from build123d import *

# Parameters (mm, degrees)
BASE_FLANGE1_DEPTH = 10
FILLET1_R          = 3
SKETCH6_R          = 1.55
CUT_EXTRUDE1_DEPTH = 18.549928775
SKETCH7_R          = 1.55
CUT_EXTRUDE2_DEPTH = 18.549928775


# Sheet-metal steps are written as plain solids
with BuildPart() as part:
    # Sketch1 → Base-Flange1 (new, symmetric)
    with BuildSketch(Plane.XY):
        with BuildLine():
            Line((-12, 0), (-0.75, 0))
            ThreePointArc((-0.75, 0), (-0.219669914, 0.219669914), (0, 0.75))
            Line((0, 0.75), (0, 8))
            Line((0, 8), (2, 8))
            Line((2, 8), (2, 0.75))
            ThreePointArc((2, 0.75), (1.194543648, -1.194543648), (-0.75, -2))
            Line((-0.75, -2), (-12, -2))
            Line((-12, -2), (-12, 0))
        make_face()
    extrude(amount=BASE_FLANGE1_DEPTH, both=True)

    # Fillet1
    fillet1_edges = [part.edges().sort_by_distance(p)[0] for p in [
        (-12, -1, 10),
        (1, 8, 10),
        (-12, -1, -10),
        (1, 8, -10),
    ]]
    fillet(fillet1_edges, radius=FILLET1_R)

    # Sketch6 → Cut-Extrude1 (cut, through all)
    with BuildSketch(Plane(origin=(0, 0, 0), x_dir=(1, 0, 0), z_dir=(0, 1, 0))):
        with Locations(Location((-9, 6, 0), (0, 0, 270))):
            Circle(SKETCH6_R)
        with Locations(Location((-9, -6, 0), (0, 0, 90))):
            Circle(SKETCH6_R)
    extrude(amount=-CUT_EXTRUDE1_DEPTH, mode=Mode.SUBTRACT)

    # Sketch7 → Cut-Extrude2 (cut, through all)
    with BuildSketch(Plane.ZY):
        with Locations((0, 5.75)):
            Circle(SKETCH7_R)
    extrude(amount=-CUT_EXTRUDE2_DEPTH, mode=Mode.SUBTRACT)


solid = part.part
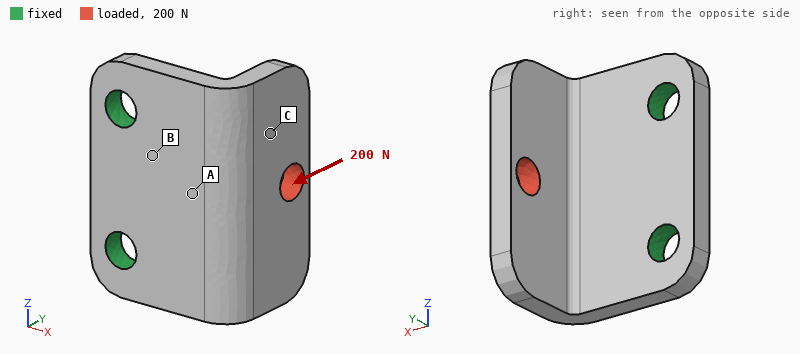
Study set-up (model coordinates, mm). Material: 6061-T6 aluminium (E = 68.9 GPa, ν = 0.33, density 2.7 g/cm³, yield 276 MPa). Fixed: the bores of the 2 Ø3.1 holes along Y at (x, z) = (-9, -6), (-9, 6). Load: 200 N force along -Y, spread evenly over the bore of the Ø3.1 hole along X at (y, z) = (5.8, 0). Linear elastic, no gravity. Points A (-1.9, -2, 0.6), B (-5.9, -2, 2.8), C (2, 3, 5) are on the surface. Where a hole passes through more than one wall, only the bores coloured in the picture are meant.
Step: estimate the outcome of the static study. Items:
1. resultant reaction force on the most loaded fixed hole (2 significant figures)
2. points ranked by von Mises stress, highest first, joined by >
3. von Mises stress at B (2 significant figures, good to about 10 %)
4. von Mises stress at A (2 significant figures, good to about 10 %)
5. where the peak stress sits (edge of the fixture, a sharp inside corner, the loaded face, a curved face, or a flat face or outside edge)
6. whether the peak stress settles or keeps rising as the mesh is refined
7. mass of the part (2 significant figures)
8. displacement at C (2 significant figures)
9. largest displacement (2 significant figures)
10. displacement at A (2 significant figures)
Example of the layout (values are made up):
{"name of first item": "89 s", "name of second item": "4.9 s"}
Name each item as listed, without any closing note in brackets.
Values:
{"resultant reaction force on the most loaded fixed hole": "100 N", "points ranked by von Mises stress, highest first, joined by >": "B > A > C", "von Mises stress at B": "77 MPa", "von Mises stress at A": "41 MPa", "where the peak stress sits": "edge of the fixture", "whether the peak stress settles or keeps rising as the mesh is refined": "keeps rising", "mass of the part": "2.1 g", "displacement at C": "0.077 mm", "largest displacement": "0.11 mm", "displacement at A": "0.035 mm"}
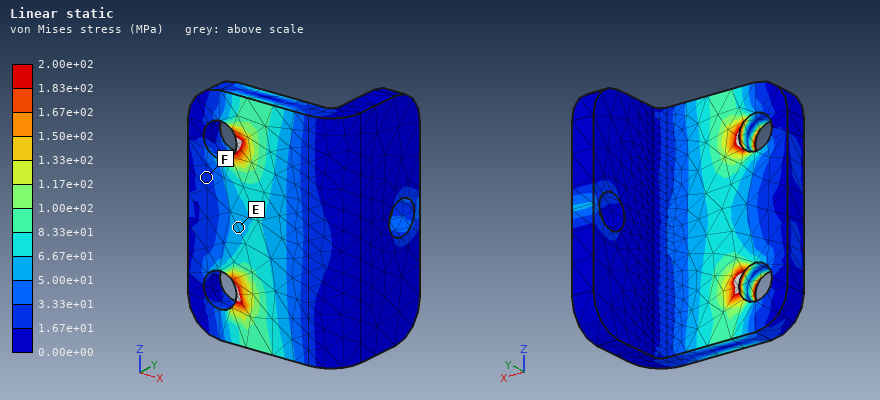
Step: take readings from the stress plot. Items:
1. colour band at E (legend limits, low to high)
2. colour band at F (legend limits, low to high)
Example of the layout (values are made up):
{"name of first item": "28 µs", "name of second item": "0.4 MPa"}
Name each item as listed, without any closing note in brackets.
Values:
{"colour band at E": "5.00e+01 to 6.67e+01 MPa", "colour band at F": "1.67e+01 to 3.33e+01 MPa"}
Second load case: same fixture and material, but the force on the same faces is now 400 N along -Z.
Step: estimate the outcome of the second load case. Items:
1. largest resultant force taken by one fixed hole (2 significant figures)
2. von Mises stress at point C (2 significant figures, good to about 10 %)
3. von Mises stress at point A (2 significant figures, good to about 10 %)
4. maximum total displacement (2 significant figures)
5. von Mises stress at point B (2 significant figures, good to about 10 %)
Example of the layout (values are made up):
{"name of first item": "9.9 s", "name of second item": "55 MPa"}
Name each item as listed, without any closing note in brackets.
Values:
{"largest resultant force taken by one fixed hole": "390 N", "von Mises stress at point C": "27 MPa", "von Mises stress at point A": "62 MPa", "maximum total displacement": "99 µm", "von Mises stress at point B": "49 MPa"}
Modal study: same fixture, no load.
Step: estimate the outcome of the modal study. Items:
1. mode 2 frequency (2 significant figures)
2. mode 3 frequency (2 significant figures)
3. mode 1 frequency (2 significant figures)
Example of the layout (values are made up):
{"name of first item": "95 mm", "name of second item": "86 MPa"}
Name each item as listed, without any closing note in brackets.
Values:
{"mode 2 frequency": "12 kHz", "mode 3 frequency": "20 kHz", "mode 1 frequency": "7100 Hz"}
